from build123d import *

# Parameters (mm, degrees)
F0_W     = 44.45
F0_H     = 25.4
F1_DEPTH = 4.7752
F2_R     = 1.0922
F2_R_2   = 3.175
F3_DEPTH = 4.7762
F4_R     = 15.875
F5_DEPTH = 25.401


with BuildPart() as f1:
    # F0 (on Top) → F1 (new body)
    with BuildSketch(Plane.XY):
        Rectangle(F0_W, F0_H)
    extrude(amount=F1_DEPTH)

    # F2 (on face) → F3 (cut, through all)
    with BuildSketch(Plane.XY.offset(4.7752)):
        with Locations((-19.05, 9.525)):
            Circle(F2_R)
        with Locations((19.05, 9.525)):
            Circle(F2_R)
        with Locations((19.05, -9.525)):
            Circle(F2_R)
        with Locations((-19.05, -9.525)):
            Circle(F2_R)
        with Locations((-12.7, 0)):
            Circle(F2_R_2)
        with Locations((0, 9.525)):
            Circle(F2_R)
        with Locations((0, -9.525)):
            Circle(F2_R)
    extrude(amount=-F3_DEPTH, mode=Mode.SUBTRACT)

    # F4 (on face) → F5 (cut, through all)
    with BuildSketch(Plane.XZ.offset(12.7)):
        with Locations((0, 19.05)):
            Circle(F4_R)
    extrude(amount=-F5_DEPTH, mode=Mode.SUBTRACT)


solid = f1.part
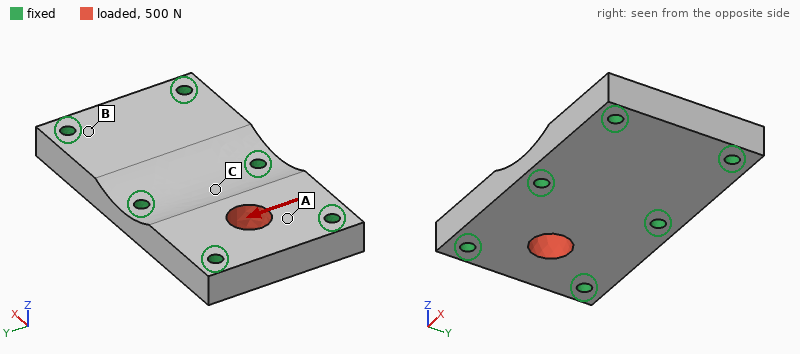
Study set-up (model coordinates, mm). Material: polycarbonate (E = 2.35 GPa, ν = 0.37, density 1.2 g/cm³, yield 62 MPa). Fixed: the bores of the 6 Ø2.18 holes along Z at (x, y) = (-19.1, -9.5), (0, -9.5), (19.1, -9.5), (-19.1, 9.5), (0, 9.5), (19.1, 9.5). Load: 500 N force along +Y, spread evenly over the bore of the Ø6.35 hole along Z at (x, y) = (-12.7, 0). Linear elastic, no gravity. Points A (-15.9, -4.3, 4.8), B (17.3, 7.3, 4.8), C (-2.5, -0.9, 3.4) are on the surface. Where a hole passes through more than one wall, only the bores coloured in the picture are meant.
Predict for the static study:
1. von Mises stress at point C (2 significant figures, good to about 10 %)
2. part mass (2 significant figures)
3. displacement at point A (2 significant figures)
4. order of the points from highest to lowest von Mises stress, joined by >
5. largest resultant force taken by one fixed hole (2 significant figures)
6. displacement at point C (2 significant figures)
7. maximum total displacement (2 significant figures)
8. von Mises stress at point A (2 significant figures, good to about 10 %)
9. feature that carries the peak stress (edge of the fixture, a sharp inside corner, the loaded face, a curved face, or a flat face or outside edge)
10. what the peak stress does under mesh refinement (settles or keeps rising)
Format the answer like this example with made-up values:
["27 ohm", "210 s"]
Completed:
["2.5 MPa", "5.7 g", "16 µm", "A > C > B", "170 N", "10 µm", "32 µm", "5.3 MPa", "edge of the fixture", "keeps rising"]
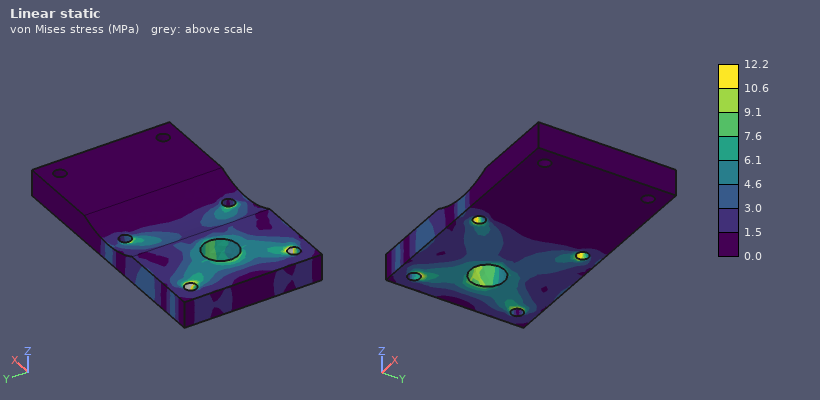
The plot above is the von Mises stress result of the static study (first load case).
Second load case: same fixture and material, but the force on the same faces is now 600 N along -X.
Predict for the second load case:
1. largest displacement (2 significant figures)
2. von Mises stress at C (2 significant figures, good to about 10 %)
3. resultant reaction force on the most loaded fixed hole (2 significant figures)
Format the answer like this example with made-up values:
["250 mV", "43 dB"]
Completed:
["49 µm", "4.3 MPa", "180 N"]
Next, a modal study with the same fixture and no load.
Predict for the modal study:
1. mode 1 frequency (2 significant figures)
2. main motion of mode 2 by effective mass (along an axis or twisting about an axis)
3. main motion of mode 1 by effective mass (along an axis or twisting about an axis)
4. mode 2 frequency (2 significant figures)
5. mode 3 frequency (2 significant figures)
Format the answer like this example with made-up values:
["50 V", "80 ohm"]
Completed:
["9200 Hz", "twisting about Y", "along Z", "10 kHz", "14 kHz"]
